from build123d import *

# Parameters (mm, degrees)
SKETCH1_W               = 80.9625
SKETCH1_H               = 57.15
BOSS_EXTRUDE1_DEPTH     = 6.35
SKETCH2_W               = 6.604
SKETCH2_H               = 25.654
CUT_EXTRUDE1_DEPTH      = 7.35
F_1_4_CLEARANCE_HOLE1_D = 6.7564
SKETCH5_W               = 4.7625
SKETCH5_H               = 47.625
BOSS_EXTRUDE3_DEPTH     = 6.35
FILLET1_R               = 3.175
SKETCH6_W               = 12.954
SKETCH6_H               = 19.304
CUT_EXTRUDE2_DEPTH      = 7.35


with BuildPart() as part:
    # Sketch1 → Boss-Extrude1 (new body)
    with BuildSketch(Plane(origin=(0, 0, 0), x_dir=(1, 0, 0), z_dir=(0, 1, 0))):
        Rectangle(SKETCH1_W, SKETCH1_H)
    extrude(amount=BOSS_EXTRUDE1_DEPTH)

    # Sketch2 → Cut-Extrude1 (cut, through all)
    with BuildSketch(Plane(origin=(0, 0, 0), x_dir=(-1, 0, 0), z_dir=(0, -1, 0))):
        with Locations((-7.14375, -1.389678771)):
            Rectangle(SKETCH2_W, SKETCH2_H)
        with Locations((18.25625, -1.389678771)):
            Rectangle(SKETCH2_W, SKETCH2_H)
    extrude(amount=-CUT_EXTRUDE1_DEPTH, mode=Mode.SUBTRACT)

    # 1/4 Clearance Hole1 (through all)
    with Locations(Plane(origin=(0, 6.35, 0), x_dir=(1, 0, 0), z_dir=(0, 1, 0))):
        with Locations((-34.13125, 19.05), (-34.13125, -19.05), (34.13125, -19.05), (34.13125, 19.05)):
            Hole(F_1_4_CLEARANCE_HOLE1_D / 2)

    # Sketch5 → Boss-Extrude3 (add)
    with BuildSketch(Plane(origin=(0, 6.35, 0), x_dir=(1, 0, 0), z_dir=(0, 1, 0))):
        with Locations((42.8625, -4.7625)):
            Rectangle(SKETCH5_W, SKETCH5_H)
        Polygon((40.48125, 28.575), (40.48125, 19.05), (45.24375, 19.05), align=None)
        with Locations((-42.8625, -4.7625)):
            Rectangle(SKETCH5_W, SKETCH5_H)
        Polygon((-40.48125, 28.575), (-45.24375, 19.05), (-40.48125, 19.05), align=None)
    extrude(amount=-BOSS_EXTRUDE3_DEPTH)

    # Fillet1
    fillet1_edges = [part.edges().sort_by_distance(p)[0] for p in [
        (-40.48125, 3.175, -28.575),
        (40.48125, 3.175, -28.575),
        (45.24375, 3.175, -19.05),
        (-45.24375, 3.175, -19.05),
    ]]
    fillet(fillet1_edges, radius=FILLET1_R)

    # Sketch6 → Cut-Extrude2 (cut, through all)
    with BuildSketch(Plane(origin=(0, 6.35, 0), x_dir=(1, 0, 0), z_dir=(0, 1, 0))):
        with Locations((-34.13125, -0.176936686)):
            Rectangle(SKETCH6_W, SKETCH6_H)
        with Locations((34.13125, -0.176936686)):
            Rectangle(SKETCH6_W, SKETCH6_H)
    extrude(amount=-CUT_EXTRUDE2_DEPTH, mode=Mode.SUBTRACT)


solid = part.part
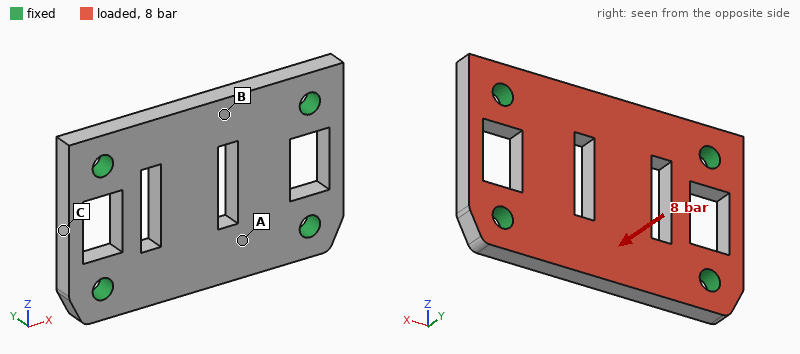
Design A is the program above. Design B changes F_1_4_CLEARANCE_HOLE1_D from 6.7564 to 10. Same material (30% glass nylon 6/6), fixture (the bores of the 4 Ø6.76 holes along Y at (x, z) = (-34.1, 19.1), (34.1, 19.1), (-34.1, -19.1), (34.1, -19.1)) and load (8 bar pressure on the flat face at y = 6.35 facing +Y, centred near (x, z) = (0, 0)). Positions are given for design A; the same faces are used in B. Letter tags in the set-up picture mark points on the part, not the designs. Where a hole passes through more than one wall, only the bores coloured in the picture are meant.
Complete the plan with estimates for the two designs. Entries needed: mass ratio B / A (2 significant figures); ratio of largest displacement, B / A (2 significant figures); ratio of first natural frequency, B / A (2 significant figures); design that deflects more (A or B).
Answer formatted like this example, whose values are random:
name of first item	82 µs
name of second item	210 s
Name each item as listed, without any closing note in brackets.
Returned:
mass ratio B / A	0.96
ratio of largest displacement, B / A	0.82
ratio of first natural frequency, B / A	1.1
design that deflects more	A
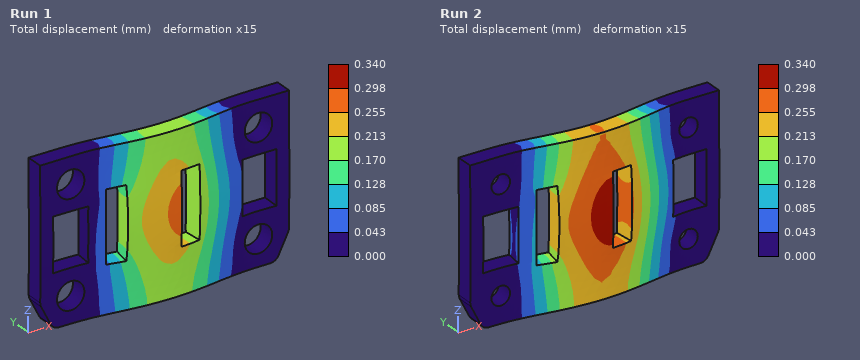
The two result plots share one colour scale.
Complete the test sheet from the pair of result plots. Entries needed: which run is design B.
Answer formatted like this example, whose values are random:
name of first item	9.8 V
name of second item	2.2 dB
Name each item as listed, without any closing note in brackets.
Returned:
which run is design B	Run 1
